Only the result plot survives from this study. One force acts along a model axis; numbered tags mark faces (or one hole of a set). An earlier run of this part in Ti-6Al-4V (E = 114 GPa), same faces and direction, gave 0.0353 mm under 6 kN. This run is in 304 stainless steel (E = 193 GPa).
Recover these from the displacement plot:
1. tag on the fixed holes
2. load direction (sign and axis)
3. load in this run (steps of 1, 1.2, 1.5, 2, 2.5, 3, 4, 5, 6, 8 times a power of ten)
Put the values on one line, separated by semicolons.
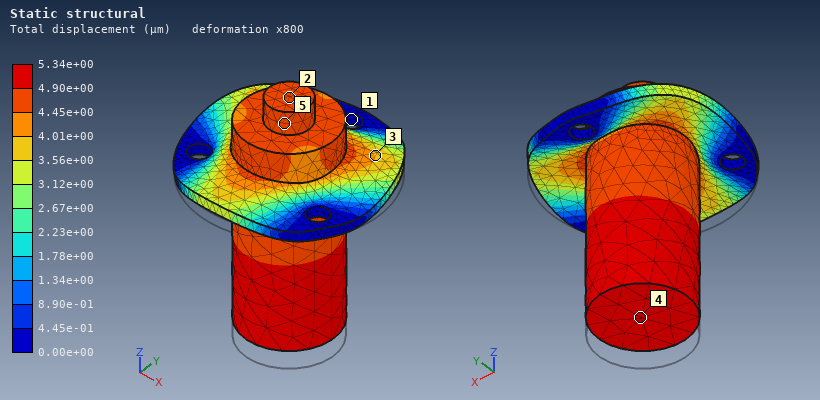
1; +Z; 1.5 kN
